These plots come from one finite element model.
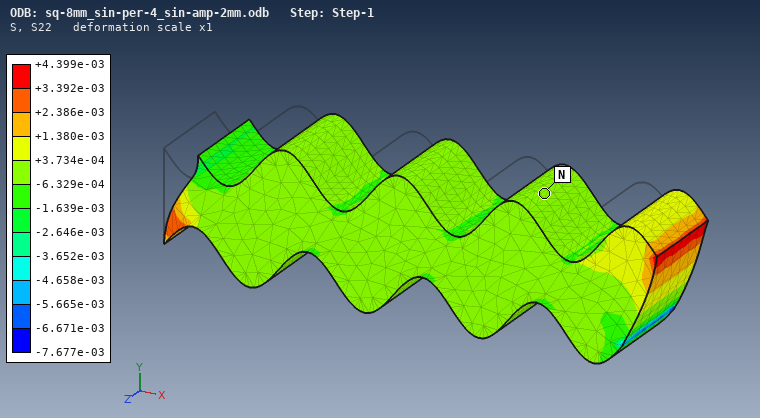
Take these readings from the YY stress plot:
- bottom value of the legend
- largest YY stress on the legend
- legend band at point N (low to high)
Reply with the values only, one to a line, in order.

-7.677e-03
+4.399e-03
-6.329e-04 to +3.734e-04
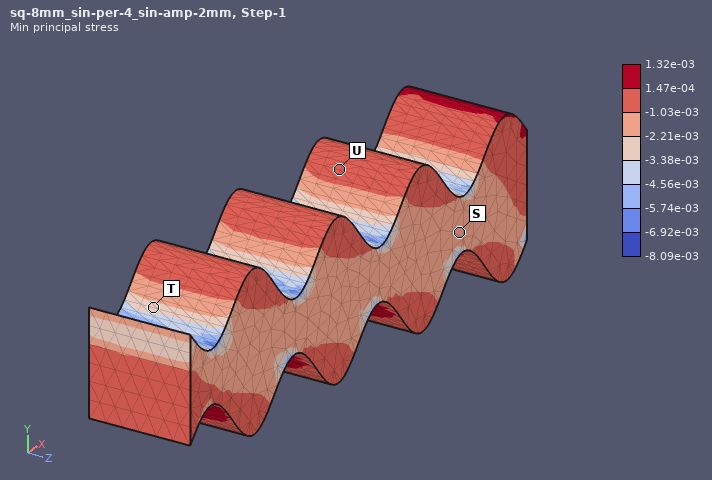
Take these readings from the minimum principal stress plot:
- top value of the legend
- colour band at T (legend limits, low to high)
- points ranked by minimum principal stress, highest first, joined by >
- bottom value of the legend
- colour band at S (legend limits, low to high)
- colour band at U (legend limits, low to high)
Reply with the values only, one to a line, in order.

1.32e-03
-3.38e-03 to -2.21e-03
U > S > T
-8.09e-03
-2.21e-03 to -1.03e-03
-1.03e-03 to 1.47e-04
